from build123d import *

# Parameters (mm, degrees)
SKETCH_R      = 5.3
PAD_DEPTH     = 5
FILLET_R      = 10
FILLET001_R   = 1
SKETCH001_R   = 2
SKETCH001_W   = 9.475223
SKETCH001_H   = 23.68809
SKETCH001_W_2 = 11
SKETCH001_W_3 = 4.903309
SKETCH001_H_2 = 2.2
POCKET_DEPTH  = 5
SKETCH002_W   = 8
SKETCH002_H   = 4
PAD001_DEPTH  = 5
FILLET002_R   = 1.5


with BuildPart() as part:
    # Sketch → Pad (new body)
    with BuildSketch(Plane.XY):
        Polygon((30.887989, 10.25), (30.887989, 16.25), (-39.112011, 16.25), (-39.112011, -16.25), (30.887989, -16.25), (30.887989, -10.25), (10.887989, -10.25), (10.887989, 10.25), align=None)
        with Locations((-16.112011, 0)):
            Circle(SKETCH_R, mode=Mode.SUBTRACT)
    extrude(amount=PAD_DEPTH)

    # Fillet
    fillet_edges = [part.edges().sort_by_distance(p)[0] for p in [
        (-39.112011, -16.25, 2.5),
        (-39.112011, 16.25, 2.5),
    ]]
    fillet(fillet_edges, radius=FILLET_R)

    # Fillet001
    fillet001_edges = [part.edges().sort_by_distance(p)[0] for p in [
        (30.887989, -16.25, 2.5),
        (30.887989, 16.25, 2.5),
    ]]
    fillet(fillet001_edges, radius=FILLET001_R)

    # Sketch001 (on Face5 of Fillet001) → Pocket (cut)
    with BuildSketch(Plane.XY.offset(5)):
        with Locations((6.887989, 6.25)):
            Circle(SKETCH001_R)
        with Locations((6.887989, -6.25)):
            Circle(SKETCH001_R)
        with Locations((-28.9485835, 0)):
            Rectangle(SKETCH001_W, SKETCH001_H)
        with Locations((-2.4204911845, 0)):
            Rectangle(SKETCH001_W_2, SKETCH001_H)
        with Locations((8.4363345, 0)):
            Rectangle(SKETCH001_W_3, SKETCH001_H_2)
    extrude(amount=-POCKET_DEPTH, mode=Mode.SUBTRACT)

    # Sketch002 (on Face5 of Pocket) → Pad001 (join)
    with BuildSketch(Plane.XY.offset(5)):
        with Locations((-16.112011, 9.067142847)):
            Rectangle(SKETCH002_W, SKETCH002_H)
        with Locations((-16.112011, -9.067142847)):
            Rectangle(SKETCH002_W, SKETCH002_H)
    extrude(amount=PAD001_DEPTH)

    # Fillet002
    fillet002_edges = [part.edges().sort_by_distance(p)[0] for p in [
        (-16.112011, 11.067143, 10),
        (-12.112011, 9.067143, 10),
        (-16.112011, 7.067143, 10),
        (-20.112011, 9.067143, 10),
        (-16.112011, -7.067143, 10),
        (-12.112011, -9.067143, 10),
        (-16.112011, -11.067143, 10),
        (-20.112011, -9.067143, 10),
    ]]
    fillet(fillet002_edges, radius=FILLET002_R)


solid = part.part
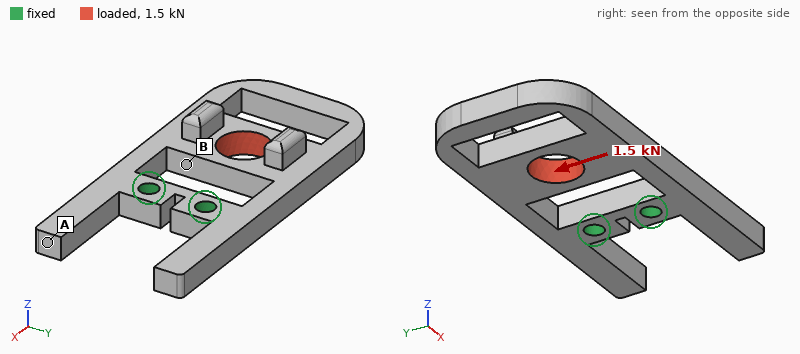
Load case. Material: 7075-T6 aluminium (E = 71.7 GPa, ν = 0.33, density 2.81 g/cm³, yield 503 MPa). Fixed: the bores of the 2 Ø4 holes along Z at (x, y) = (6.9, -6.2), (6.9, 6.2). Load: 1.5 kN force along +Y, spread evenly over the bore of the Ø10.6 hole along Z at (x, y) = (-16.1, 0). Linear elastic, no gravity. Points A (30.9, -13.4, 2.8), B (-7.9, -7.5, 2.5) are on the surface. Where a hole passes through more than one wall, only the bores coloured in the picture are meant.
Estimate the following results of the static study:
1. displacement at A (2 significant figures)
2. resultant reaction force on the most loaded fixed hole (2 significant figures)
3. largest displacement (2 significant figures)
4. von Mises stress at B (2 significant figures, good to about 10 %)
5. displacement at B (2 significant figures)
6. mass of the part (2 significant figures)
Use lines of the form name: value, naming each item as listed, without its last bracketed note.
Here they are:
displacement at A: 0.12 mm
resultant reaction force on the most loaded fixed hole: 1.2 kN
largest displacement: 0.30 mm
von Mises stress at B: 74 MPa
displacement at B: 0.18 mm
mass of the part: 18 g
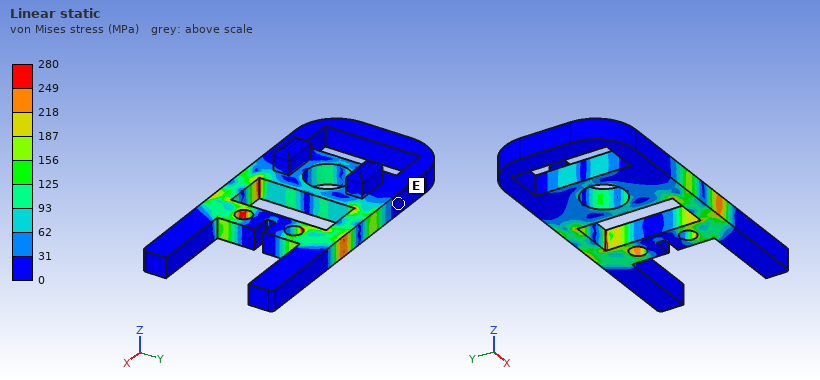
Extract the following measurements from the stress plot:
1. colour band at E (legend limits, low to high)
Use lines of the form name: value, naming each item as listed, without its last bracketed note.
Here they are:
colour band at E: 0 to 31 MPa
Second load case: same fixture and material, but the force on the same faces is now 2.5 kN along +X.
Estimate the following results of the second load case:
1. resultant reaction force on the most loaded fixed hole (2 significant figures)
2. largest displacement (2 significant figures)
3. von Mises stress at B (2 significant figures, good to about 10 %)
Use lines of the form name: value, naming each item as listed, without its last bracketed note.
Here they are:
resultant reaction force on the most loaded fixed hole: 1.3 kN
largest displacement: 68 µm
von Mises stress at B: 42 MPa
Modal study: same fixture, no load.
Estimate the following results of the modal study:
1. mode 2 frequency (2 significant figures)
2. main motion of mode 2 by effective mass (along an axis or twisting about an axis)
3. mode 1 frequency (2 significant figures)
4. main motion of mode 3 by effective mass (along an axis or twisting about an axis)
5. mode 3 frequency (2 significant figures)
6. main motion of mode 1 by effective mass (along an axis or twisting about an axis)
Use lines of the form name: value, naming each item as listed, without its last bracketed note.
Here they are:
mode 2 frequency: 3500 Hz
main motion of mode 2 by effective mass: along Y
mode 1 frequency: 1200 Hz
main motion of mode 3 by effective mass: twisting about X
mode 3 frequency: 4100 Hz
main motion of mode 1 by effective mass: along Z
